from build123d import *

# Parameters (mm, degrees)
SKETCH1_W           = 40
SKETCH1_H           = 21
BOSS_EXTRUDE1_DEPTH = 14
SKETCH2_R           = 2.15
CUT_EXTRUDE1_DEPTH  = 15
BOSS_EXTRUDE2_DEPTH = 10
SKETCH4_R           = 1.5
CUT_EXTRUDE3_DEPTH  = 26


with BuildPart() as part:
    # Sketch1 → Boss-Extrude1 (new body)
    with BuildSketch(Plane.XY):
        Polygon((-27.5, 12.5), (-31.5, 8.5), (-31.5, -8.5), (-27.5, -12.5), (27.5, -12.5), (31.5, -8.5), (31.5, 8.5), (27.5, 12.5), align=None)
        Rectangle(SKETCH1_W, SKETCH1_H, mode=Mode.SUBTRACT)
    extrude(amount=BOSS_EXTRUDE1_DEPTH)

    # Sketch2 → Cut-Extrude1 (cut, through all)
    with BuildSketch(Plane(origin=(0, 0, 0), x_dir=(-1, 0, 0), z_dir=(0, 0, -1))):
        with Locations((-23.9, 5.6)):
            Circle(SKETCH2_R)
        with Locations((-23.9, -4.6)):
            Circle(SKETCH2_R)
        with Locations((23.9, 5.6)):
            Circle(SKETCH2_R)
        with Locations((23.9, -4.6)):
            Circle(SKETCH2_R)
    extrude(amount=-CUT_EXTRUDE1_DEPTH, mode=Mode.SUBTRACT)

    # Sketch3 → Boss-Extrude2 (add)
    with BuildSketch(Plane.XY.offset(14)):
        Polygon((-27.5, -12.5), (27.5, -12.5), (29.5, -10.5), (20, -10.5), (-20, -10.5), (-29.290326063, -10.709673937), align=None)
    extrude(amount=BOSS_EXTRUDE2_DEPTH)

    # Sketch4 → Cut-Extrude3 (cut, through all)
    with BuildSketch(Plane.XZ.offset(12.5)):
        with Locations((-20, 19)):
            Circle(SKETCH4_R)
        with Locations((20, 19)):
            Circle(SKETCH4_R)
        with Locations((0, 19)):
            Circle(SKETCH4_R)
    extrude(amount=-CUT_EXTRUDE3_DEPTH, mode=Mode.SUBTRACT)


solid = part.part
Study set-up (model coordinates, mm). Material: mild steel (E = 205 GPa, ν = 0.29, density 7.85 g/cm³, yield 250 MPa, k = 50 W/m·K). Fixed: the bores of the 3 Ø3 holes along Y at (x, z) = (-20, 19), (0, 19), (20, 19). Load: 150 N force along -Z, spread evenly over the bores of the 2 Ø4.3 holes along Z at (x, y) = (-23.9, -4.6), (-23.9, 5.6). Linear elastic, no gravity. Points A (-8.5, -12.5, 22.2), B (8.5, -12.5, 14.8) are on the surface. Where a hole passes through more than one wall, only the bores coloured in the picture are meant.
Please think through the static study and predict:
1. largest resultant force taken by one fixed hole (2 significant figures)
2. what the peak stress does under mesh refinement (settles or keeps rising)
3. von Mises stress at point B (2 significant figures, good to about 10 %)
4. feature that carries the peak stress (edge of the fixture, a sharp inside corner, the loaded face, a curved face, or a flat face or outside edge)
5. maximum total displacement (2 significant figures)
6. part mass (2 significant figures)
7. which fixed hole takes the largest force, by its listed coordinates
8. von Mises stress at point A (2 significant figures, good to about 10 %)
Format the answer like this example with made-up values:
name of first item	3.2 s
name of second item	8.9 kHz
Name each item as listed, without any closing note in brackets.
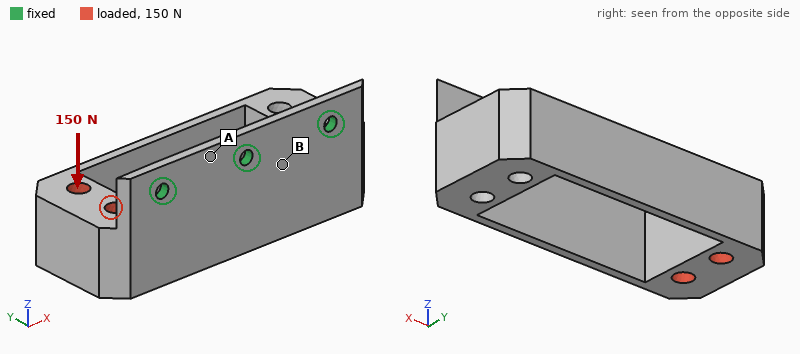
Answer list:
largest resultant force taken by one fixed hole	170 N
what the peak stress does under mesh refinement	keeps rising
von Mises stress at point B	23 MPa
feature that carries the peak stress	edge of the fixture
maximum total displacement	66 µm
part mass	79 g
which fixed hole takes the largest force, by its listed coordinates	(-20, 19)
von Mises stress at point A	7.9 MPa
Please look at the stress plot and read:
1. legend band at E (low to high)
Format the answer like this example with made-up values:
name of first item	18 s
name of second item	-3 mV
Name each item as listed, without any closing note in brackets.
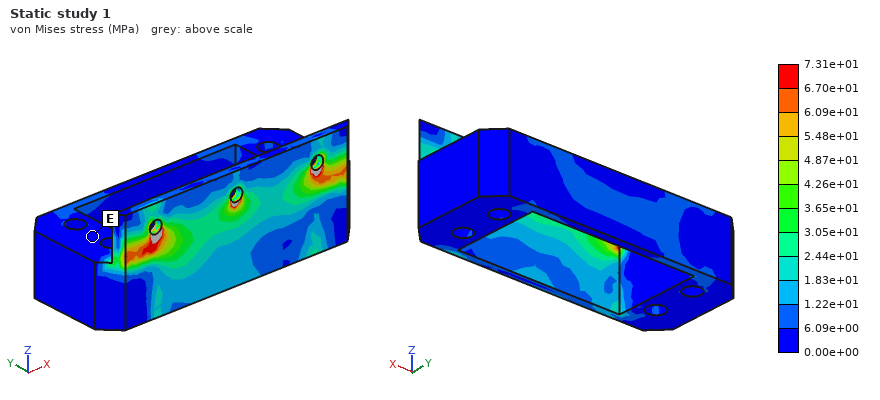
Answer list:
legend band at E	0.00e+00 to 6.09e+00 MPa
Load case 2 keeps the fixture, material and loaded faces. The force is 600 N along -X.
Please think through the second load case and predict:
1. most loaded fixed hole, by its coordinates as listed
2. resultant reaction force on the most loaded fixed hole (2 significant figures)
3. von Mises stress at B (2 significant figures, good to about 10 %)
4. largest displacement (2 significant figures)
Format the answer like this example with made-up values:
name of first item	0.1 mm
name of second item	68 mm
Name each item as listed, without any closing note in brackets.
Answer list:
most loaded fixed hole, by its coordinates as listed	(-20, 19)
resultant reaction force on the most loaded fixed hole	310 N
von Mises stress at B	23 MPa
largest displacement	92 µm
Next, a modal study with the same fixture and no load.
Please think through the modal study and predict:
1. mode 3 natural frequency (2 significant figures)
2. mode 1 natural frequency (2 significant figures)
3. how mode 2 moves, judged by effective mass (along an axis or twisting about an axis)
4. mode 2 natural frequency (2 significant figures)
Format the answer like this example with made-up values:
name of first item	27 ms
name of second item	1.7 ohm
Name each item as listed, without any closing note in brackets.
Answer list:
mode 3 natural frequency	3400 Hz
mode 1 natural frequency	1000 Hz
how mode 2 moves, judged by effective mass	along X
mode 2 natural frequency	1700 Hz
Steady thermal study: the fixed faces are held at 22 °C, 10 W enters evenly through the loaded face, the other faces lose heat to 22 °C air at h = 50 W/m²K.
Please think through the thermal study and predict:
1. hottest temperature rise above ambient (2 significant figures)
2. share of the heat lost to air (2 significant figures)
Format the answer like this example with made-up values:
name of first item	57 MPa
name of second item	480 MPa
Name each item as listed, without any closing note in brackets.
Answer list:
hottest temperature rise above ambient	39 K
share of the heat lost to air	45 %
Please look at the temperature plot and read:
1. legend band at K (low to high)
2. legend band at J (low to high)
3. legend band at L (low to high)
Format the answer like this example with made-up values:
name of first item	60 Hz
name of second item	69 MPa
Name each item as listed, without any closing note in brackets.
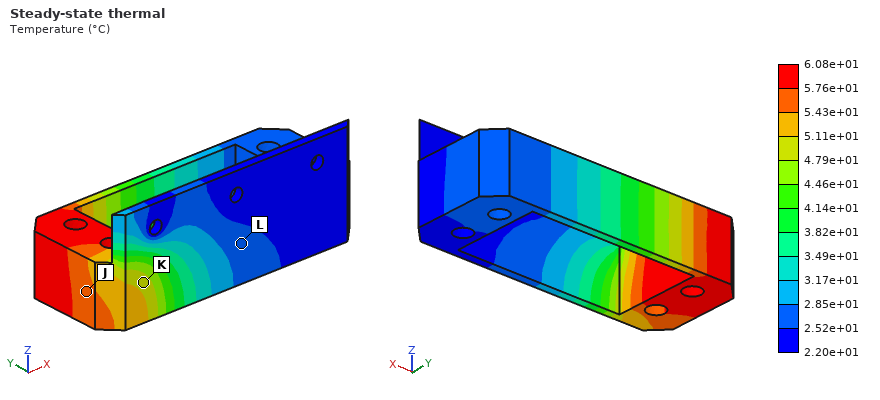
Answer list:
legend band at K	4.79e+01 to 5.11e+01 °C
legend band at J	5.43e+01 to 5.76e+01 °C
legend band at L	2.52e+01 to 2.85e+01 °C
